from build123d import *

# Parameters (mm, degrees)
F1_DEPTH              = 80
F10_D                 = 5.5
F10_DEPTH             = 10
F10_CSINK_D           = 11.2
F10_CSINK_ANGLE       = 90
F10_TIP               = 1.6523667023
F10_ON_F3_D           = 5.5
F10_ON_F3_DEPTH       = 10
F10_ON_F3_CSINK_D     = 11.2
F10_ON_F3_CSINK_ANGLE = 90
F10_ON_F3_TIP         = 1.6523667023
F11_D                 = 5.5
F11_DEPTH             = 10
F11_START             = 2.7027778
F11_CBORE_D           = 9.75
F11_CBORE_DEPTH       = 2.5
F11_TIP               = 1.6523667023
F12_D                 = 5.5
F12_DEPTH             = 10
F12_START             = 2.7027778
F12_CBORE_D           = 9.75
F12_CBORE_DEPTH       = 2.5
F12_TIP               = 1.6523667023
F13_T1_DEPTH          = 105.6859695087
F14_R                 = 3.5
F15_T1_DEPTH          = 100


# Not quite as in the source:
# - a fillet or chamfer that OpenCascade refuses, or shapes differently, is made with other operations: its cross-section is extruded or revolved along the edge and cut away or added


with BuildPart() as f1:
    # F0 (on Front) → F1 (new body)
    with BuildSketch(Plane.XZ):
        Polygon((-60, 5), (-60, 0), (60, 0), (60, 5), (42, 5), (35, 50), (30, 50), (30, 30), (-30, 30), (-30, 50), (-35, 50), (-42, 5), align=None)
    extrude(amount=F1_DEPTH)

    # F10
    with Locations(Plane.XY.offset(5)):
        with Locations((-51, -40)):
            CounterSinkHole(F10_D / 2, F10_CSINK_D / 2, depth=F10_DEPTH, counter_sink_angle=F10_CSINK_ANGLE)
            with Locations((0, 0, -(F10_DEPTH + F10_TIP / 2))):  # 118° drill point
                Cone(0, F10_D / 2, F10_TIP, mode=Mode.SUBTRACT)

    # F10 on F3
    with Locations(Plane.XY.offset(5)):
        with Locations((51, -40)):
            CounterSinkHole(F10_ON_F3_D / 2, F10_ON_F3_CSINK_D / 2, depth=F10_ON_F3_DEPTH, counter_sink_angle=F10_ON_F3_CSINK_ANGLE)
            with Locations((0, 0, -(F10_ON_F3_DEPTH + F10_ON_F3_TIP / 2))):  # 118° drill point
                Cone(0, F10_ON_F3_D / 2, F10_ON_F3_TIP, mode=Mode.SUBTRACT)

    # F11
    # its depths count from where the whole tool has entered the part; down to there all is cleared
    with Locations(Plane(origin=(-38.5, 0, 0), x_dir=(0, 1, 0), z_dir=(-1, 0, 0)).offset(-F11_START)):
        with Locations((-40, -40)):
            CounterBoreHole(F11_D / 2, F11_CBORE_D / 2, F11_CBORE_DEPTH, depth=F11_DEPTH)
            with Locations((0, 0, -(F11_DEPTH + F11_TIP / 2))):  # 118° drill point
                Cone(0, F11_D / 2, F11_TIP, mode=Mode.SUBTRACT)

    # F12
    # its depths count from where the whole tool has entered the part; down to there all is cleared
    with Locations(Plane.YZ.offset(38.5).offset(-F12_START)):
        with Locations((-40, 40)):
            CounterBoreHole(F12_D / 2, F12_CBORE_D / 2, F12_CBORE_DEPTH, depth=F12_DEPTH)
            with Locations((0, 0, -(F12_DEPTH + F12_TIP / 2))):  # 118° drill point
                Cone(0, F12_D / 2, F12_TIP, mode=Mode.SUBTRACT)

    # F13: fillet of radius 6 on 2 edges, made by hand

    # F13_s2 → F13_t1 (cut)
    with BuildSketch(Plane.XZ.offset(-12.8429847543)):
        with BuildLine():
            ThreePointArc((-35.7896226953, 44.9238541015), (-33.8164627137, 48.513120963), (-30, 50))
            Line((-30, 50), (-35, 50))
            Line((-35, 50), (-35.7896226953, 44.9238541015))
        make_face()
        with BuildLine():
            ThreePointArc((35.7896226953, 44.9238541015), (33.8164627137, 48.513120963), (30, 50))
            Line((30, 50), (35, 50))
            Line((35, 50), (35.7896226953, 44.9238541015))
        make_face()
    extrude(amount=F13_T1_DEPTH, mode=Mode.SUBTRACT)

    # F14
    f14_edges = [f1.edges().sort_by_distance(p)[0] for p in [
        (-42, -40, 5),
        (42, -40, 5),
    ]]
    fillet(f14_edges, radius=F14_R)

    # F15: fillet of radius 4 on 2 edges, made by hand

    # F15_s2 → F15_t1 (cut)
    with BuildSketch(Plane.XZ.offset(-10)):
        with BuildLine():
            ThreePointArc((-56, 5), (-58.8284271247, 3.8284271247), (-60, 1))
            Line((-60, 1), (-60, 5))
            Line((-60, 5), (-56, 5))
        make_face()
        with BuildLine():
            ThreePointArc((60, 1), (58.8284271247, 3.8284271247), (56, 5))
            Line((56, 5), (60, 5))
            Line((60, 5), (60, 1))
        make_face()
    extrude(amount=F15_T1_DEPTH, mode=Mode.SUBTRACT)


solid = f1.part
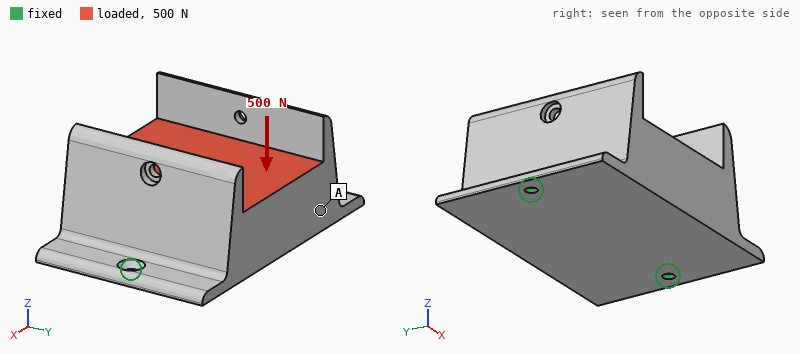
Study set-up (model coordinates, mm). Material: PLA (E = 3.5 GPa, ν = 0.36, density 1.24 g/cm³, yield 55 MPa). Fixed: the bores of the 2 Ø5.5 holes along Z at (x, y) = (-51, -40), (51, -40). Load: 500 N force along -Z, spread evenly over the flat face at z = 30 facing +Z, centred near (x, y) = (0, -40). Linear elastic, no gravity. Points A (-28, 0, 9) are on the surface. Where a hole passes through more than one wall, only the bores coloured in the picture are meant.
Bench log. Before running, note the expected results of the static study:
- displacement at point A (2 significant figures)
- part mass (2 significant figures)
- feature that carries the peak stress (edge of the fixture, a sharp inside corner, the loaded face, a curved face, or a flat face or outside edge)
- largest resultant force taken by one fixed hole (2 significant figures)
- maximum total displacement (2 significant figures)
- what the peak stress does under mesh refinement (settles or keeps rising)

68 µm
280 g
edge of the fixture
350 N
72 µm
keeps rising
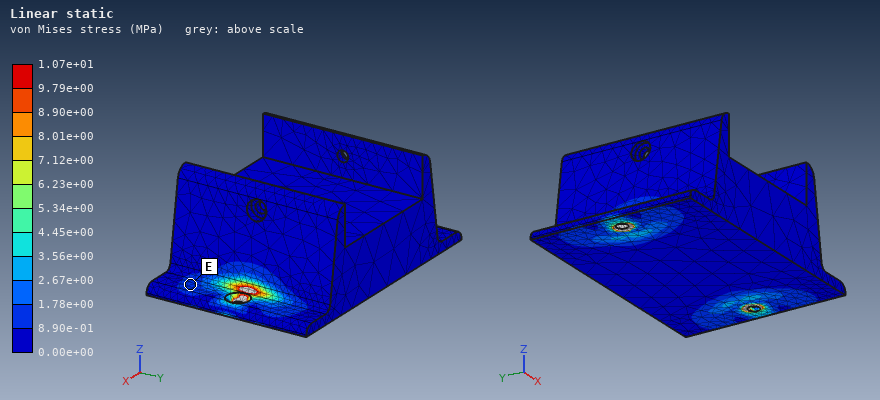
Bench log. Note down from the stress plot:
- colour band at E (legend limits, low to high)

8.90e-01 to 1.78e+00 MPa
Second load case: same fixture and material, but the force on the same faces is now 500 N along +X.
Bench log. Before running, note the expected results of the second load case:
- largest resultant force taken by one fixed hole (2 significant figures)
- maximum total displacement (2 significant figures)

290 N
44 µm
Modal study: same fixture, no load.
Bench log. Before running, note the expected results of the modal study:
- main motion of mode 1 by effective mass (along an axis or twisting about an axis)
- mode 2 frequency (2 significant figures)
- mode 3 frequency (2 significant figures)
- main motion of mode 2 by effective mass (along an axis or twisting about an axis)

along Y
830 Hz
1300 Hz
along Z
